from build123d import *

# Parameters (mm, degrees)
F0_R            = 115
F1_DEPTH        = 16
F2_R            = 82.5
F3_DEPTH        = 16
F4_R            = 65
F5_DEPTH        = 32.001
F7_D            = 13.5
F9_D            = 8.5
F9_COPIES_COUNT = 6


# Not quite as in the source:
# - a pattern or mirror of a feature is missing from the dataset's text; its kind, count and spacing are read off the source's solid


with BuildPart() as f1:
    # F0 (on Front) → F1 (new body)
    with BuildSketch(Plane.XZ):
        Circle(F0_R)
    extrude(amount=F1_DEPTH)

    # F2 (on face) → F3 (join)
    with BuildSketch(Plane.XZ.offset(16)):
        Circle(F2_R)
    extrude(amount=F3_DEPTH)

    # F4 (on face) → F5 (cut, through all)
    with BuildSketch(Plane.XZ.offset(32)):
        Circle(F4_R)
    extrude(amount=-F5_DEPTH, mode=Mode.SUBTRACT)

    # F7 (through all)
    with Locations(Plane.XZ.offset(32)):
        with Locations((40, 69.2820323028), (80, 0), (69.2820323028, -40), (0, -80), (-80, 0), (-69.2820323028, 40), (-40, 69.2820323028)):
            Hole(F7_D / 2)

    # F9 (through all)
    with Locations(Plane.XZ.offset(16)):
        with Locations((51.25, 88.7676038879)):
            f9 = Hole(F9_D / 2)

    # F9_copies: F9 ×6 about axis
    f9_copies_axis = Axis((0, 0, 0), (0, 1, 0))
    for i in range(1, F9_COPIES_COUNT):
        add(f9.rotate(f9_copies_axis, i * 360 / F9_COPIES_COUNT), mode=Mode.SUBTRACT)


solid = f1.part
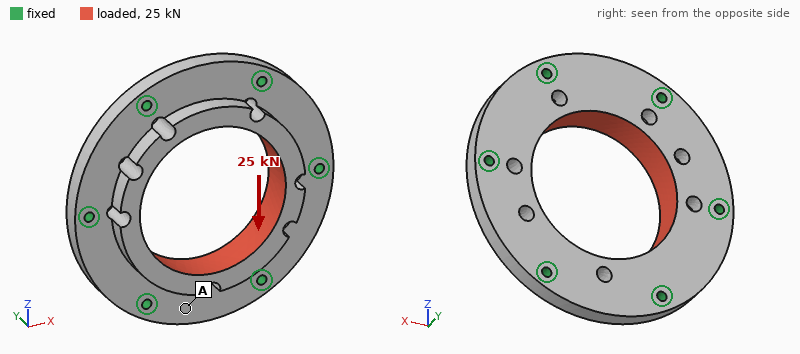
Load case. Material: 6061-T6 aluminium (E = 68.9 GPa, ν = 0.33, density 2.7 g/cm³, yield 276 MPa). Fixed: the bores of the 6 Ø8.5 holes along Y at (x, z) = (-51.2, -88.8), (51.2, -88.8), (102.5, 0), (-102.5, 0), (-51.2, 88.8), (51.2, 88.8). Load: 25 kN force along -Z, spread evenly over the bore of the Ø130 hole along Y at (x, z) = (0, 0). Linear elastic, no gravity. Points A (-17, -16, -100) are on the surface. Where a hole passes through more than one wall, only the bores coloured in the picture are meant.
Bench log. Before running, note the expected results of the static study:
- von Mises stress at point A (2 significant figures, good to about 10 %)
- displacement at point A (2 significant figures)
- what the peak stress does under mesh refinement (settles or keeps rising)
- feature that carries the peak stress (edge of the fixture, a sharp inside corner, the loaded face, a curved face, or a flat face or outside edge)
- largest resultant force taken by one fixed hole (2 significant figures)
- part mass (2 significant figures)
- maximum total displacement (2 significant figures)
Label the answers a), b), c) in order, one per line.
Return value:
a) 3.1 MPa
b) 6.0 µm
c) keeps rising
d) a sharp inside corner
e) 4.8 kN
f) 1.5 kg
g) 15 µm
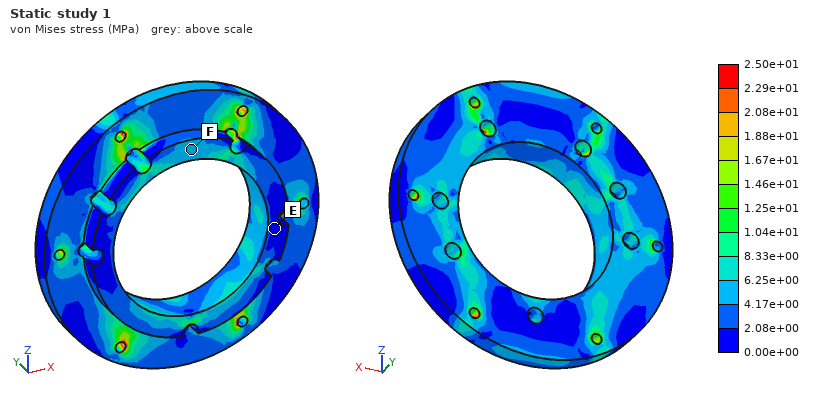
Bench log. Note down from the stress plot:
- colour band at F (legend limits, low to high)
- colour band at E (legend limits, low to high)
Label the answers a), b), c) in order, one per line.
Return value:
a) 4.17e+00 to 6.25e+00 MPa
b) 0.00e+00 to 2.08e+00 MPa
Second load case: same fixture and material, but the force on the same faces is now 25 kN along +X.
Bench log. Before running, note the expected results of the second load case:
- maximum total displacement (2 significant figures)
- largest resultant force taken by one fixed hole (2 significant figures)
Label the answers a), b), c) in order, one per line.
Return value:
a) 14 µm
b) 4.8 kN
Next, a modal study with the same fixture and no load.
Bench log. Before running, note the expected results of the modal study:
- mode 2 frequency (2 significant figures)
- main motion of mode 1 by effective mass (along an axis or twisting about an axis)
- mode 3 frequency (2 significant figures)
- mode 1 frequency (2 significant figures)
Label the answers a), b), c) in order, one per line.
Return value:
a) 6000 Hz
b) along Y
c) 6000 Hz
d) 5100 Hz
